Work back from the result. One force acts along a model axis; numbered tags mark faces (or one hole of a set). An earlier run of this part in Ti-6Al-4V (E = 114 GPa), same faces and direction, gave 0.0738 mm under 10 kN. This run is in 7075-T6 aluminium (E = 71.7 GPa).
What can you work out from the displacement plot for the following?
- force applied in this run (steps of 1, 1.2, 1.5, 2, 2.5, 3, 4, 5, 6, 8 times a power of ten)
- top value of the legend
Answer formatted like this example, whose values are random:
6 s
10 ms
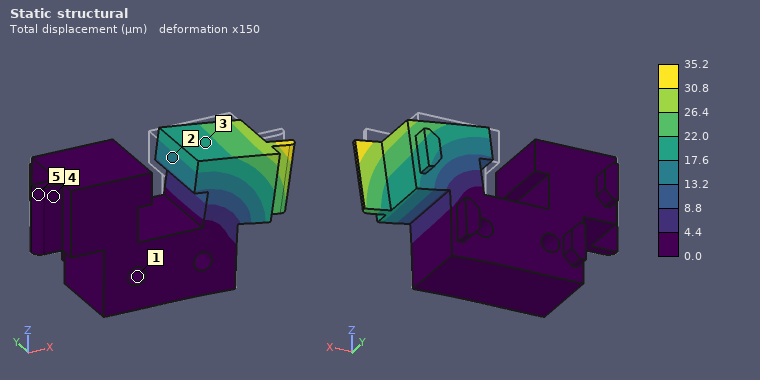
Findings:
3 kN
35.2 µm
